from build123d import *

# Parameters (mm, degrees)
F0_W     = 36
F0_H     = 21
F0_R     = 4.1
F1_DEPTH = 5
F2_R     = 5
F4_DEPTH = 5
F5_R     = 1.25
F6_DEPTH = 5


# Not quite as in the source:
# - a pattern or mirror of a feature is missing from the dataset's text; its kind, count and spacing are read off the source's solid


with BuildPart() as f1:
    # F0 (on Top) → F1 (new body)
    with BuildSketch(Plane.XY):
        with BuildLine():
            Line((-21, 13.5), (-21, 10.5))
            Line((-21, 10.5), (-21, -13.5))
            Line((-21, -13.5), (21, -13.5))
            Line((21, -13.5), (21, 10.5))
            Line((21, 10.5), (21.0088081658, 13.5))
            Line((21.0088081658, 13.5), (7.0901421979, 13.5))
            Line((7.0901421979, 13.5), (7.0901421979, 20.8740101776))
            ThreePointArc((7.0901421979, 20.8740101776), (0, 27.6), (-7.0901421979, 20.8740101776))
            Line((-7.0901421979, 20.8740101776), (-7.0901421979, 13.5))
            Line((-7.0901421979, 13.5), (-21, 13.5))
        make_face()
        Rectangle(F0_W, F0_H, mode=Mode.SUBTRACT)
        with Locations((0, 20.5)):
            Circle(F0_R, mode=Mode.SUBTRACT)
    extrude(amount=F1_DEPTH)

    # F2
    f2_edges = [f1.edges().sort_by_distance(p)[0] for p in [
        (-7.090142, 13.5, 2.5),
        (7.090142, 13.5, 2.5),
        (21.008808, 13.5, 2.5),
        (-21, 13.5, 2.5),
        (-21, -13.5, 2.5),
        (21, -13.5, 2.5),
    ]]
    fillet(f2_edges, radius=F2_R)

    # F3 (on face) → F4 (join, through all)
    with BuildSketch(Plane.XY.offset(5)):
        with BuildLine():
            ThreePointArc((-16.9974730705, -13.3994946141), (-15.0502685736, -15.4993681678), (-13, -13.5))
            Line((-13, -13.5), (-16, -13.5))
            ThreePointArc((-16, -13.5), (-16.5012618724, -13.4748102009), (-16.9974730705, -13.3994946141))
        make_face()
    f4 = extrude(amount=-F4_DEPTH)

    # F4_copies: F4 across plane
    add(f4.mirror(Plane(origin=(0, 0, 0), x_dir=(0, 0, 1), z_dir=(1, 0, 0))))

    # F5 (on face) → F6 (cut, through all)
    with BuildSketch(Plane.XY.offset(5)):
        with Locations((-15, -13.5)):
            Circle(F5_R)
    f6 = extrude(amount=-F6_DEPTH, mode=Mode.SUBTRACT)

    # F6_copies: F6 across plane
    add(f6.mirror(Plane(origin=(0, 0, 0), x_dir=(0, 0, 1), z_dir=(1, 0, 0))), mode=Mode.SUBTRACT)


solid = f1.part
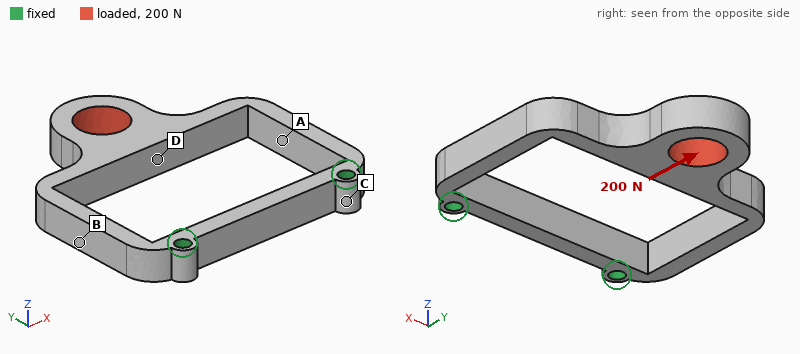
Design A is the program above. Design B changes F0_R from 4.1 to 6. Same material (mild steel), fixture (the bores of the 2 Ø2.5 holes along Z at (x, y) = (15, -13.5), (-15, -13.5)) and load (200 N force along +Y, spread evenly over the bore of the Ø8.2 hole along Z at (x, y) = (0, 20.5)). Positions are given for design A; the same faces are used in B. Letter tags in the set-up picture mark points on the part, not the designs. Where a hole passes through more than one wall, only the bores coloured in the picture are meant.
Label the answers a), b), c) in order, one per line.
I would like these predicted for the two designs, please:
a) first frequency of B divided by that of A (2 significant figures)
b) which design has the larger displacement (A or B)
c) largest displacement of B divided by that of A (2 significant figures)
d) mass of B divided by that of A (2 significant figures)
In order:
a) 1.2
b) B
c) 1.3
d) 0.88
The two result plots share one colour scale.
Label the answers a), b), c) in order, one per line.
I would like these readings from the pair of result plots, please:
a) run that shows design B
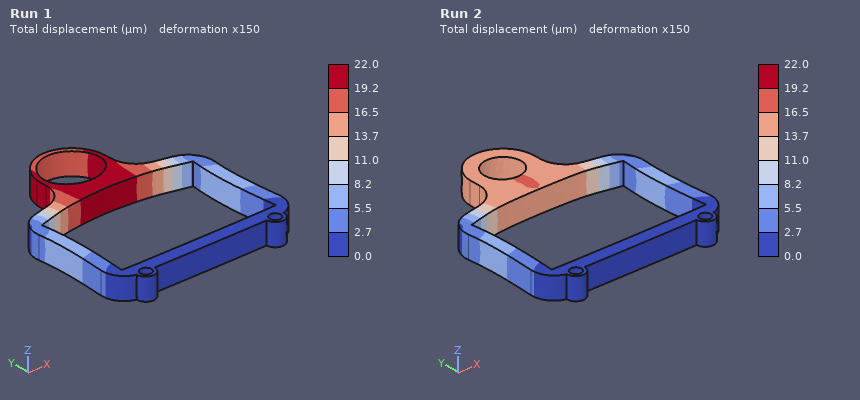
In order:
a) Run 1
